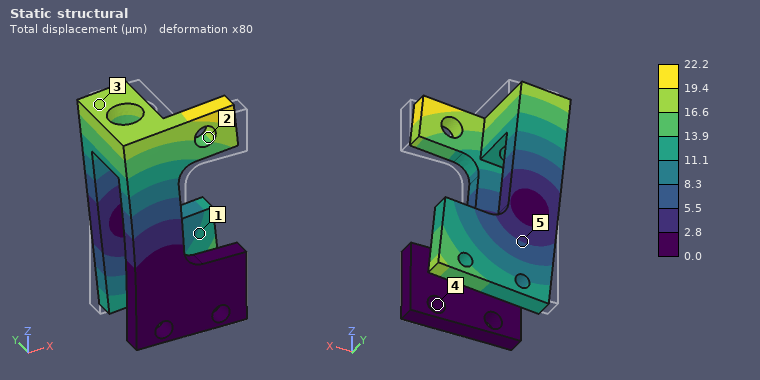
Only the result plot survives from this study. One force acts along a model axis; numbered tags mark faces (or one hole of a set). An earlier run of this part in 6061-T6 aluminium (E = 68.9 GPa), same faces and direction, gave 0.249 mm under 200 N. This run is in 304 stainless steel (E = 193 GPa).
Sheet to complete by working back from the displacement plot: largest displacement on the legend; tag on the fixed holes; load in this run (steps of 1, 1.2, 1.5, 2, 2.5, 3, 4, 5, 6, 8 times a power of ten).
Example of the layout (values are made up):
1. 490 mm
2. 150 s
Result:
1. 22.2 µm
2. 4
3. 50 N
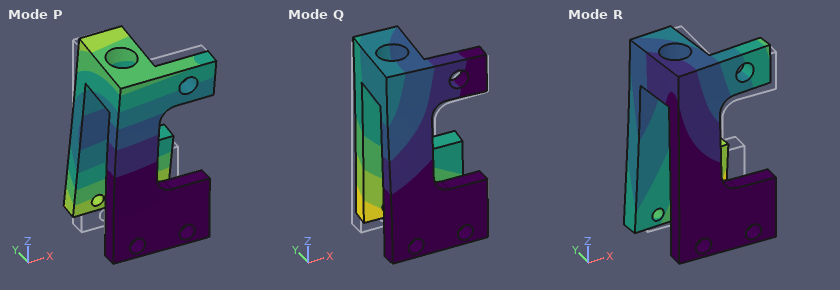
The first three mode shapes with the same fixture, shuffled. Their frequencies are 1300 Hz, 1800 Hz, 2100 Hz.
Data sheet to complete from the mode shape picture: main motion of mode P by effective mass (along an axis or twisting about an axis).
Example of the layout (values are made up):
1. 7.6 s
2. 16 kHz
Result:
1. along Z
